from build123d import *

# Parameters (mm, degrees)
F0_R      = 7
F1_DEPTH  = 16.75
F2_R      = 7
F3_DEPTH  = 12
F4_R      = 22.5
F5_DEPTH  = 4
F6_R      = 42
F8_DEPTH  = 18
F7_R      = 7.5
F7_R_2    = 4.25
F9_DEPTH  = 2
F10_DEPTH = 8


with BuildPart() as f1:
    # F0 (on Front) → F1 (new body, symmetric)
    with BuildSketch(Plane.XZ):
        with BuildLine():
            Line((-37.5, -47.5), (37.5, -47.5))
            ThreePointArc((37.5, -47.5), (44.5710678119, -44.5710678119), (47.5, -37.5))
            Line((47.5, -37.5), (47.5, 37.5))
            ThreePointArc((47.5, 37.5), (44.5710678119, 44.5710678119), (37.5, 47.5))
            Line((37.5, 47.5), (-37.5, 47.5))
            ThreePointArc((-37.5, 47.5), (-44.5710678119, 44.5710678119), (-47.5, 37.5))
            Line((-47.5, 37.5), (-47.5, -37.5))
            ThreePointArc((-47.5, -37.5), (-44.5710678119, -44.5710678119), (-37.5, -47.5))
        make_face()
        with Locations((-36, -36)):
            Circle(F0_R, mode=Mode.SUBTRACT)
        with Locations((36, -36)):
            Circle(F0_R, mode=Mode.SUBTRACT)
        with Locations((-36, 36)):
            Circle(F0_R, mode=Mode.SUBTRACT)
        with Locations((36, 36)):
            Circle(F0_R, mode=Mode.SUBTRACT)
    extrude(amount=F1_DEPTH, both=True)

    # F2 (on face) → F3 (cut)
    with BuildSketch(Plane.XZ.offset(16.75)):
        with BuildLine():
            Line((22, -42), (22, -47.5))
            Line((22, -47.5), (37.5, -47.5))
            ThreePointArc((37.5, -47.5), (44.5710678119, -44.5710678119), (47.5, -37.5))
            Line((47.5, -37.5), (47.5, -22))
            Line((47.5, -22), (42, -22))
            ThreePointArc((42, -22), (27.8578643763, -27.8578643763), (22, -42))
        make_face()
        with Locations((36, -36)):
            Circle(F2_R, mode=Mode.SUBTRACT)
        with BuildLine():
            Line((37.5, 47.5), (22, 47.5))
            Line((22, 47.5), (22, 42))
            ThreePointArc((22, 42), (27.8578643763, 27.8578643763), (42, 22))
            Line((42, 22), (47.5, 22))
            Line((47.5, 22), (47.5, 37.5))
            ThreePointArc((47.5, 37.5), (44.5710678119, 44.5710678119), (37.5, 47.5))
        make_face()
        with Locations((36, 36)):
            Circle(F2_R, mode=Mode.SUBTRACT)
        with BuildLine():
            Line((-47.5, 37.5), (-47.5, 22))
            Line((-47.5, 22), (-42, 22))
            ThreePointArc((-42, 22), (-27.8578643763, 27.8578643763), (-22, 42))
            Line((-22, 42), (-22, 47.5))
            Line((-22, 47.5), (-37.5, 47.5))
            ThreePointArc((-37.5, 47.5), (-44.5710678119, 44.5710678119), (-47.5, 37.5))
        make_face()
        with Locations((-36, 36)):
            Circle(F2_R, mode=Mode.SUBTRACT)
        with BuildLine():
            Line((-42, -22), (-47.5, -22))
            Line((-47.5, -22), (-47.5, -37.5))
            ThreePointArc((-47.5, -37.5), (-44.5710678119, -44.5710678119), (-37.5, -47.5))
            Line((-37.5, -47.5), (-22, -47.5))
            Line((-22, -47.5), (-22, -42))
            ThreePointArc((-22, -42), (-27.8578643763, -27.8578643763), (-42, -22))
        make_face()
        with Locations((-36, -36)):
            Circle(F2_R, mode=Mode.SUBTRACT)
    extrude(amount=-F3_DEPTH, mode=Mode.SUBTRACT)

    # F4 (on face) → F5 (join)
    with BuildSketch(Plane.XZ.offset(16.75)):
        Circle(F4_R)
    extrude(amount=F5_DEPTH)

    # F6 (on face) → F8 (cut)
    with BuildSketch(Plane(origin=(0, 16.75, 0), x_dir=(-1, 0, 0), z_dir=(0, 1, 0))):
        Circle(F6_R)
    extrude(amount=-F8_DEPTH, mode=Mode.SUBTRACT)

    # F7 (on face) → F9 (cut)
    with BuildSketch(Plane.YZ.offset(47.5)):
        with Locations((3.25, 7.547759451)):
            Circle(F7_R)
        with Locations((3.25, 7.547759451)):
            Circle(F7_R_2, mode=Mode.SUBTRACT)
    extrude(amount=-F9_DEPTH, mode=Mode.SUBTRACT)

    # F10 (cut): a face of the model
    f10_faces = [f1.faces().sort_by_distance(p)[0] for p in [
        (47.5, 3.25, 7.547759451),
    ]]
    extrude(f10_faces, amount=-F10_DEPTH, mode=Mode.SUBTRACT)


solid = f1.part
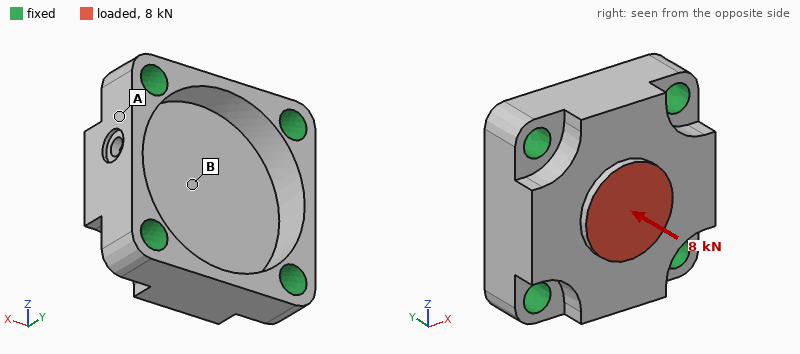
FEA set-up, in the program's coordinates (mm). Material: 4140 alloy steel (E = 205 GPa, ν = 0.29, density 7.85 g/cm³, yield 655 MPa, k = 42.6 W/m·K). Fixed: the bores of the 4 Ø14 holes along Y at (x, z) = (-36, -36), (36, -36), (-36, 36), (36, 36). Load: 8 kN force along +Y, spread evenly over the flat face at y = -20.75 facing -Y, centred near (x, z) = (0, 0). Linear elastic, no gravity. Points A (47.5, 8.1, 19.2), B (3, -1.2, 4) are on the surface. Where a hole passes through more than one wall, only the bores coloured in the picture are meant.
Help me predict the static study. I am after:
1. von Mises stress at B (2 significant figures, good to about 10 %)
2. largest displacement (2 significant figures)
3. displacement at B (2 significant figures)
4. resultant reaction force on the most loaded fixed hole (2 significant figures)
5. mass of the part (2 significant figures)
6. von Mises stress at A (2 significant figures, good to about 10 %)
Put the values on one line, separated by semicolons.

12 MPa; 5.3 µm; 5.1 µm; 2.8 kN; 1.3 kg; 4.0 MPa
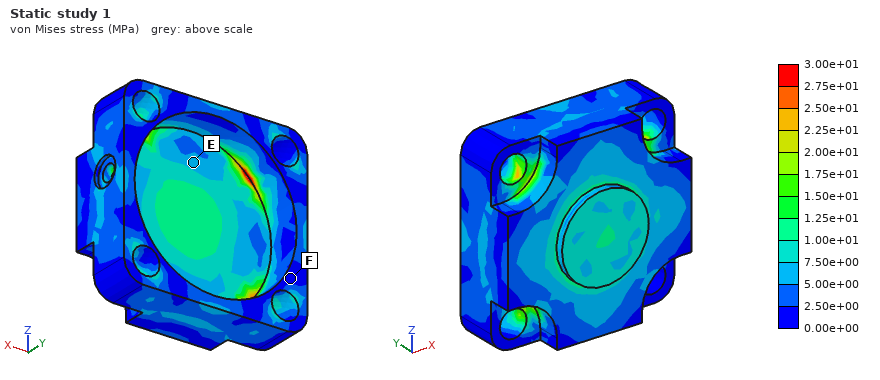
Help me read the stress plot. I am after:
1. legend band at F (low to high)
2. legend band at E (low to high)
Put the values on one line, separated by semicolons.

0.00e+00 to 2.50e+00 MPa; 5.00e+00 to 7.50e+00 MPa
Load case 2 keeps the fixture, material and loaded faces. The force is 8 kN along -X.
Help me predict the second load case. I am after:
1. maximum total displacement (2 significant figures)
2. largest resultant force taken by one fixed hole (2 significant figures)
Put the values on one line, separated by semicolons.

2.7 µm; 2.5 kN
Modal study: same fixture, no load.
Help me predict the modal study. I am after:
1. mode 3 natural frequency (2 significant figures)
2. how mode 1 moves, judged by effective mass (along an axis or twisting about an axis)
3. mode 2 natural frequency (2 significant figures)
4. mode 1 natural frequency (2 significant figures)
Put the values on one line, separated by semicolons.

14 kHz; along Y; 14 kHz; 10 kHz
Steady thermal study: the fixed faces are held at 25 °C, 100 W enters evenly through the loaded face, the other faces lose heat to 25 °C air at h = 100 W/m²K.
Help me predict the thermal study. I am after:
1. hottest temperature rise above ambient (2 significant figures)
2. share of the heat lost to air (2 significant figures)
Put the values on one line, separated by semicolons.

47 K; 35 %
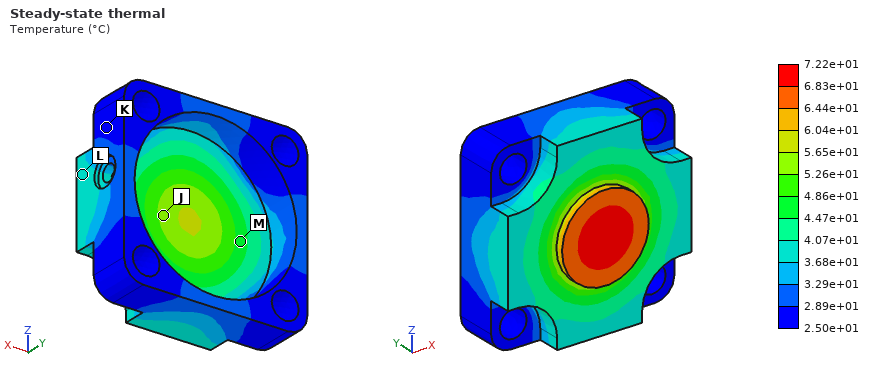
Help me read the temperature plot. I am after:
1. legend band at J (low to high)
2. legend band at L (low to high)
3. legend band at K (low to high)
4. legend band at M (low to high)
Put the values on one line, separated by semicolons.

5.26e+01 to 5.65e+01 °C; 3.68e+01 to 4.07e+01 °C; 2.50e+01 to 2.89e+01 °C; 4.47e+01 to 4.86e+01 °C
